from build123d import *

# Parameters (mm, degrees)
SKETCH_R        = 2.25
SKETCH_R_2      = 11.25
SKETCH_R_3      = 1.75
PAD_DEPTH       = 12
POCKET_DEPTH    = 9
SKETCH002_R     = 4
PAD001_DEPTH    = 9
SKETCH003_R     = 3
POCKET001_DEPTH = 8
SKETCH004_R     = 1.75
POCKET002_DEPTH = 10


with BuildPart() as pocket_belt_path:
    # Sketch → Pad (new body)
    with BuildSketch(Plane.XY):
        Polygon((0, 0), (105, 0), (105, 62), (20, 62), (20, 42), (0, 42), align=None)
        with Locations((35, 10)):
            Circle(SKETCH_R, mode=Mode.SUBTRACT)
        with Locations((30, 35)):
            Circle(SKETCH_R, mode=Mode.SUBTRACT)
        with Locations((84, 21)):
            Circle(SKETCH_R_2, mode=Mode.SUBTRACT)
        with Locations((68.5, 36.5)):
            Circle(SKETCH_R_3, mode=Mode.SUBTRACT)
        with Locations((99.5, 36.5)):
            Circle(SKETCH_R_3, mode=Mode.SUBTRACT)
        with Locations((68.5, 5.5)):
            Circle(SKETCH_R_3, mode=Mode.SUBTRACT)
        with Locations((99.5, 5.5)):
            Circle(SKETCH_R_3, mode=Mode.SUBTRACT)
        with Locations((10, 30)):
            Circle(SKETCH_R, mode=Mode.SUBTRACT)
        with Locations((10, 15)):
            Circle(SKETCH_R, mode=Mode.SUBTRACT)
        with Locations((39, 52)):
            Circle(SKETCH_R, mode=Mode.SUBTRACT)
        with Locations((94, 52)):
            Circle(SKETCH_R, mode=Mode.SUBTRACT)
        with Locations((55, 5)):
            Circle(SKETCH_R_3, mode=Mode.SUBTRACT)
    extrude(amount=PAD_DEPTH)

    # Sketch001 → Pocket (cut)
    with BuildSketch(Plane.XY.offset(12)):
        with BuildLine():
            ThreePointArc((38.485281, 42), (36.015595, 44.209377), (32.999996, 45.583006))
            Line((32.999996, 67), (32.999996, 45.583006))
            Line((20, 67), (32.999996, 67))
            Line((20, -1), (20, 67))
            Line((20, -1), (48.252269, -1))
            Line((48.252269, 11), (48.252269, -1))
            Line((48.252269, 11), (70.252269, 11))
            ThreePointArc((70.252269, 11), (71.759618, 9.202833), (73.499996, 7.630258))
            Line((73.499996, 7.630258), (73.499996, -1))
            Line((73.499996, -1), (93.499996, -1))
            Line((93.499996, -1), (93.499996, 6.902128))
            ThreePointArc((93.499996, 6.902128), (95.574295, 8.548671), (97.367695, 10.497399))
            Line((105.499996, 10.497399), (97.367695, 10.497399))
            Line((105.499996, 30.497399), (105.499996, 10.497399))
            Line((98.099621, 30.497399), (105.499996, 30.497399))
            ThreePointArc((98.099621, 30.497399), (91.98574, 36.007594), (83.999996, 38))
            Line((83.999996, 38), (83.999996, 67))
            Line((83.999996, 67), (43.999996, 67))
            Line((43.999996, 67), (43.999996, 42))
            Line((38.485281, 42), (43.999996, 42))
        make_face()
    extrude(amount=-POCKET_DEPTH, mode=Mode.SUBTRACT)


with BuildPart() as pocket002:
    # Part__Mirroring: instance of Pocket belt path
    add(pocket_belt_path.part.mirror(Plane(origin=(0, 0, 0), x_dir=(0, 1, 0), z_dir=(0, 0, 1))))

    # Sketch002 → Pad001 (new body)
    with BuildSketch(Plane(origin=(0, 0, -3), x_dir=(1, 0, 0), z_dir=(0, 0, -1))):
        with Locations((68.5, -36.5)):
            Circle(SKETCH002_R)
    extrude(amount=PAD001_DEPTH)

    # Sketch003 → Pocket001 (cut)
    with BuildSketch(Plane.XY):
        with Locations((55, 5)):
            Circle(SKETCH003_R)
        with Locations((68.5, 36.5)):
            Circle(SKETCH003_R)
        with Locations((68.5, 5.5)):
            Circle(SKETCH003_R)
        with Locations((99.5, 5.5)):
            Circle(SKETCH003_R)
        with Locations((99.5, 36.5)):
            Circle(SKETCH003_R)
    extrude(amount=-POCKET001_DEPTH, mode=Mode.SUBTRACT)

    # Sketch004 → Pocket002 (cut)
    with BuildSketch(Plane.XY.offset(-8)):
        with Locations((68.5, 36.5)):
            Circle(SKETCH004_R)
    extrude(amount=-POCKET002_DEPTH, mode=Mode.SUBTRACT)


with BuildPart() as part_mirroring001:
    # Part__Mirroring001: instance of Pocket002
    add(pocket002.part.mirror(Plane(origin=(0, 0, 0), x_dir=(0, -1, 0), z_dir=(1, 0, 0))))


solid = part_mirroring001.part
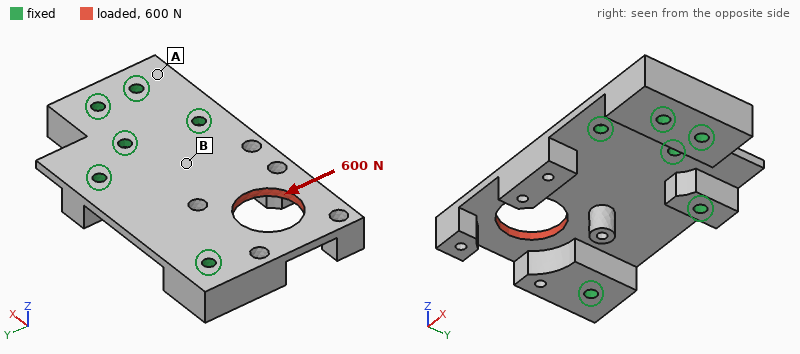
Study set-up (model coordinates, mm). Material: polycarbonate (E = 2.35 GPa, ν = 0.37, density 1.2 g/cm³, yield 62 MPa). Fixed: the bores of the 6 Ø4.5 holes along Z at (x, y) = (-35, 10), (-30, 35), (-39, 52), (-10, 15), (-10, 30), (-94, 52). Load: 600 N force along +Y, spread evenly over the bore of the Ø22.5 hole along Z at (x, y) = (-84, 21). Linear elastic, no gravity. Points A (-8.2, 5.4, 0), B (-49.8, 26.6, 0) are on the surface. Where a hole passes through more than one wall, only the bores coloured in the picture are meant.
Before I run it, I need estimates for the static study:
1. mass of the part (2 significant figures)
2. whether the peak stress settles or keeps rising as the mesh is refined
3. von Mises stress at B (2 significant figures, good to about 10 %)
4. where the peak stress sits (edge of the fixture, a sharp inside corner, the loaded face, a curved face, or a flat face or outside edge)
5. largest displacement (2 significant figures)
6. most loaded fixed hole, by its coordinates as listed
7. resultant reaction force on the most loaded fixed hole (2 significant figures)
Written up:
40 g
keeps rising
2.6 MPa
a sharp inside corner
0.22 mm
(-94, 52)
430 N
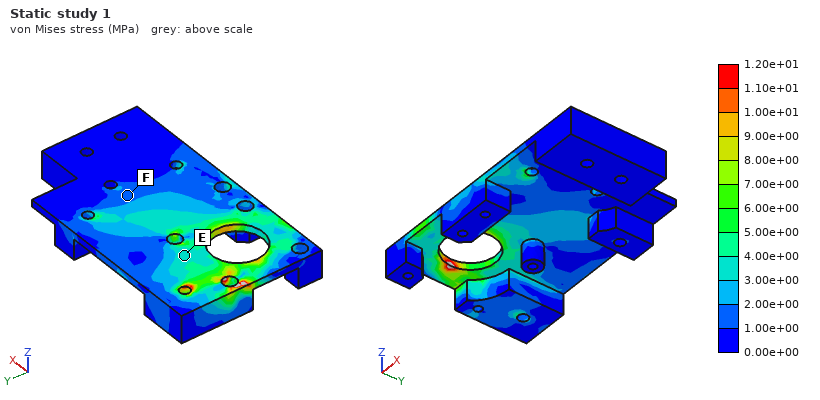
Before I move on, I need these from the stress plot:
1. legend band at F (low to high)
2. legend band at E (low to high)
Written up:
1.00e+00 to 2.00e+00 MPa
3.00e+00 to 4.00e+00 MPa
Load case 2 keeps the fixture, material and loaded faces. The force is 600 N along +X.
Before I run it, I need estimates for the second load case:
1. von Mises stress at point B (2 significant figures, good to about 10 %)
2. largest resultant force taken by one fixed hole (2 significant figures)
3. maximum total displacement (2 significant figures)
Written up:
2.0 MPa
210 N
0.17 mm
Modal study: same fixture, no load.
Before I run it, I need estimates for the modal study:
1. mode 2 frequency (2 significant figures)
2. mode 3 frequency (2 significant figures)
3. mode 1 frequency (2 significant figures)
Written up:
910 Hz
1600 Hz
450 Hz
